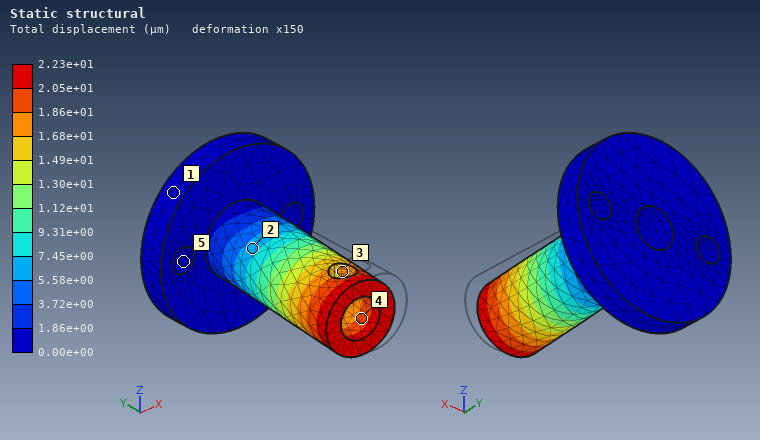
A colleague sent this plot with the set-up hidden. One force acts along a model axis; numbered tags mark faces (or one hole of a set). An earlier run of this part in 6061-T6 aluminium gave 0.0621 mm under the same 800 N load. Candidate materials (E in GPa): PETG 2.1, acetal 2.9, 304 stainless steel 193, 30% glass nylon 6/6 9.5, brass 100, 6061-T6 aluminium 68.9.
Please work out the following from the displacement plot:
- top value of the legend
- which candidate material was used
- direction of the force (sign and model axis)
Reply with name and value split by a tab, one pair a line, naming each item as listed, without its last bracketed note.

top value of the legend	2.23e+01 µm
which candidate material was used	304 stainless steel
direction of the force	-X
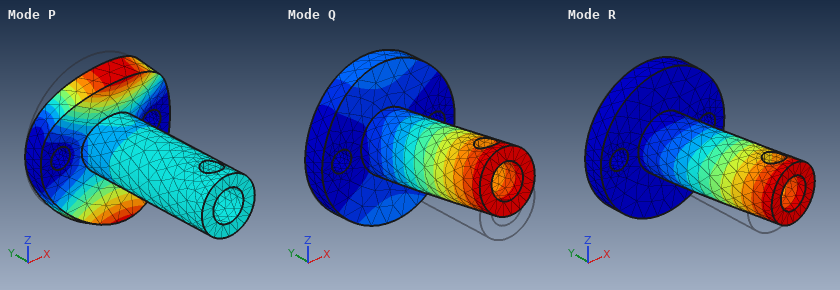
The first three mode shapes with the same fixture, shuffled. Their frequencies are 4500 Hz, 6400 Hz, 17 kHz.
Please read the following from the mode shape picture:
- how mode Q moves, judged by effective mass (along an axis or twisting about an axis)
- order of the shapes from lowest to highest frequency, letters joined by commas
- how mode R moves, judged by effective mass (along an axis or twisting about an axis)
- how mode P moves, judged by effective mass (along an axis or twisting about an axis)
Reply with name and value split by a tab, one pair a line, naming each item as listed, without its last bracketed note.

how mode Q moves, judged by effective mass	along Z
order of the shapes from lowest to highest frequency, letters joined by commas	Q, R, P
how mode R moves, judged by effective mass	along X
how mode P moves, judged by effective mass	along Y
